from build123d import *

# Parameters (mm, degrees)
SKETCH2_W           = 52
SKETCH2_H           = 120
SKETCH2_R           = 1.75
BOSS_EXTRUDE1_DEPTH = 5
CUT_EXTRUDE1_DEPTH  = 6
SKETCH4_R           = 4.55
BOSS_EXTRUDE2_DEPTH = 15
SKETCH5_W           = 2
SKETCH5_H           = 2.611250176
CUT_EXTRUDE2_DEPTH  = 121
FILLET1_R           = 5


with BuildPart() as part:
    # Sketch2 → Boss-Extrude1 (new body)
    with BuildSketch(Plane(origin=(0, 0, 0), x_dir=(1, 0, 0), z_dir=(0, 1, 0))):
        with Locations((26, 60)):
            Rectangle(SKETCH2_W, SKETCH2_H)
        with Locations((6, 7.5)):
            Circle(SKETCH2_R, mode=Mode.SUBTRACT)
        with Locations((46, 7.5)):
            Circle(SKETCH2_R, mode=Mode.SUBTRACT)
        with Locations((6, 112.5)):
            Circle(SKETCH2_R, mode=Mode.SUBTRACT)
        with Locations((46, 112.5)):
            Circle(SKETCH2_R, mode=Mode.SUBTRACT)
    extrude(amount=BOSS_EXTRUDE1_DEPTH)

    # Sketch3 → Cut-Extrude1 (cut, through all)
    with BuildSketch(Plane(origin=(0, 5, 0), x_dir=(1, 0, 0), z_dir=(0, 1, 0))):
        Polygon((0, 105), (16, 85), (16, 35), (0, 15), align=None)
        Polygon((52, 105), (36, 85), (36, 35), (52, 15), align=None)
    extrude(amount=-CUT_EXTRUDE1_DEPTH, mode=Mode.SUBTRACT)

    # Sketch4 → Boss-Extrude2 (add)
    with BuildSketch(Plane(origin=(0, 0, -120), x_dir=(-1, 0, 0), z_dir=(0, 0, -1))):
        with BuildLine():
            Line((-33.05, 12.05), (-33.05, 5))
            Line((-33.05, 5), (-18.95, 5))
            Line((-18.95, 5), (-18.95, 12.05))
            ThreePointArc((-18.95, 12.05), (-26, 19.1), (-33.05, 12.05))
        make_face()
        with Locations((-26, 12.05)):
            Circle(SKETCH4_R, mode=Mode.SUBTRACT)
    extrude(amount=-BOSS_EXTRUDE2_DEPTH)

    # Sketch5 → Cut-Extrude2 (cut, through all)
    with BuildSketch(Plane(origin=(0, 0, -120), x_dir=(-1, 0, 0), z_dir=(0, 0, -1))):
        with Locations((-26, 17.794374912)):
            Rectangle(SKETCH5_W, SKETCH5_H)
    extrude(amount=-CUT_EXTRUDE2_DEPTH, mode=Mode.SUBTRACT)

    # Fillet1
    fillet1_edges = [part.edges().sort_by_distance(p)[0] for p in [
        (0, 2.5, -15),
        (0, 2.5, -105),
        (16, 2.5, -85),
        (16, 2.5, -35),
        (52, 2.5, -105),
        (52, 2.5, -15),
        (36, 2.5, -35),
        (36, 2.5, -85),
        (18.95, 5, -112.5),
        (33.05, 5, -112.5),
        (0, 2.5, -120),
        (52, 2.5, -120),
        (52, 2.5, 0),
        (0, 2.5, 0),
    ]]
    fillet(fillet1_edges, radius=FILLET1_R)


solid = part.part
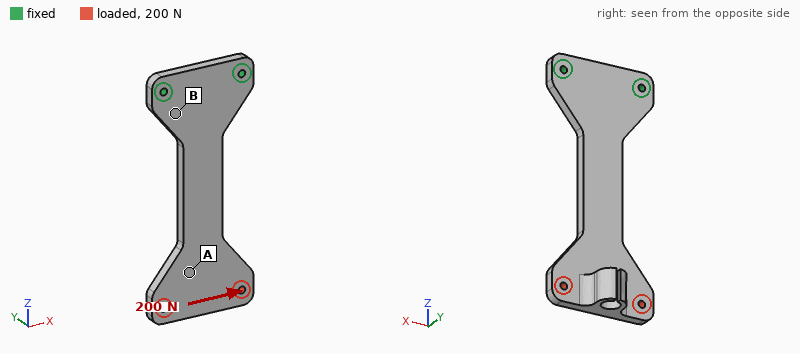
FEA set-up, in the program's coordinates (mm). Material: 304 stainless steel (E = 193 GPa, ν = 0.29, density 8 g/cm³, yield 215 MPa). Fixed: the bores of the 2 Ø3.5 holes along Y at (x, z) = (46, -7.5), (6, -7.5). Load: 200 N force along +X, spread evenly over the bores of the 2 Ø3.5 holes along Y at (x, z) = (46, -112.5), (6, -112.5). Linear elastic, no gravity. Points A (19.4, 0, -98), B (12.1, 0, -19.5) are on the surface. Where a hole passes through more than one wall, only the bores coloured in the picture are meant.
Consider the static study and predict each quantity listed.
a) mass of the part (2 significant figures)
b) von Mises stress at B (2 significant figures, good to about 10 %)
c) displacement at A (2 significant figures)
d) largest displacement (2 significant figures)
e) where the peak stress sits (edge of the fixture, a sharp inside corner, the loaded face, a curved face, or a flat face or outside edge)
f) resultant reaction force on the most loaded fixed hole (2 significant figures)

170 g
11 MPa
53 µm
81 µm
a curved face
530 N
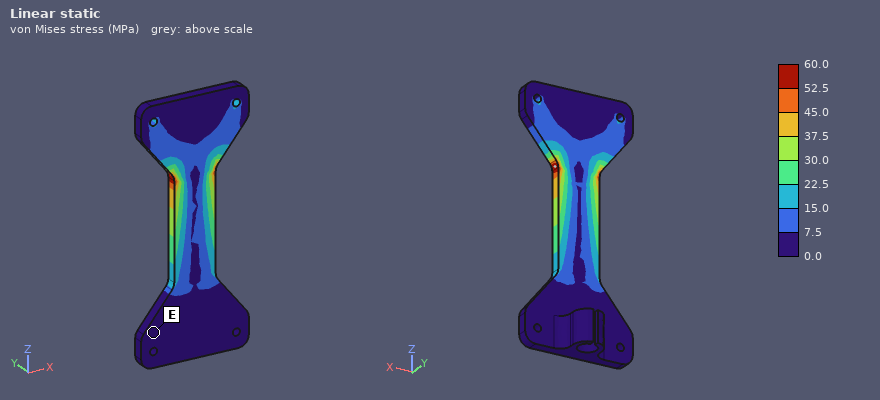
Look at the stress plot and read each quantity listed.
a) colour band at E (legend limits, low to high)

0.0 to 7.5 MPa
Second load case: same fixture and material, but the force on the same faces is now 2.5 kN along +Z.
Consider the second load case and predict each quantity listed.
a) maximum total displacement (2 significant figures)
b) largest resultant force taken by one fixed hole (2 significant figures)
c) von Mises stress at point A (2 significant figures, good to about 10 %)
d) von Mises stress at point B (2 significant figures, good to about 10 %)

15 µm
1.3 kN
13 MPa
18 MPa
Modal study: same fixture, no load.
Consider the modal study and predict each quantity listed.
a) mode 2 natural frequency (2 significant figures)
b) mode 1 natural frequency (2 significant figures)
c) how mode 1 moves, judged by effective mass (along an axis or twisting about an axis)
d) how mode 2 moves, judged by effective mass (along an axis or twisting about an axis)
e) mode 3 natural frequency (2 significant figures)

1000 Hz
220 Hz
along Y
along X
1300 Hz
